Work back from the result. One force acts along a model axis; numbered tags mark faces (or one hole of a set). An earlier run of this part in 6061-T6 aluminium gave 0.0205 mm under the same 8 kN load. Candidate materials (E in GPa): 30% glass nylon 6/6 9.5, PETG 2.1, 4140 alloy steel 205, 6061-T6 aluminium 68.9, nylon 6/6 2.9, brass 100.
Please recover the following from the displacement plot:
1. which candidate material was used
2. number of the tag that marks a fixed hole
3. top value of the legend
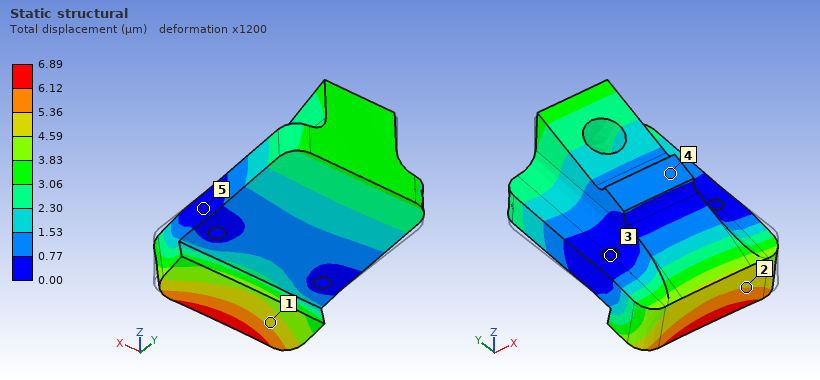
4140 alloy steel
3
6.89 µm
